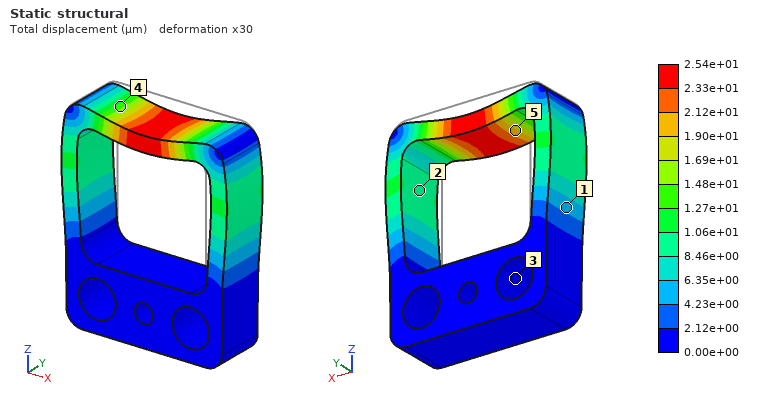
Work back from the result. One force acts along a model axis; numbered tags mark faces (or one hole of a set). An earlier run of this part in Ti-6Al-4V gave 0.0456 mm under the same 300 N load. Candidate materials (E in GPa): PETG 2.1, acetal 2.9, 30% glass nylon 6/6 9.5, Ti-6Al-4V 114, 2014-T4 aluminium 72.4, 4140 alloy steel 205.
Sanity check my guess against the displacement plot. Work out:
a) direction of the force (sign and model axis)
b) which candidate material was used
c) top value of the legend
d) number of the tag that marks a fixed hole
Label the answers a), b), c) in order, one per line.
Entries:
a) -Z
b) 4140 alloy steel
c) 2.54e+01 µm
d) 3
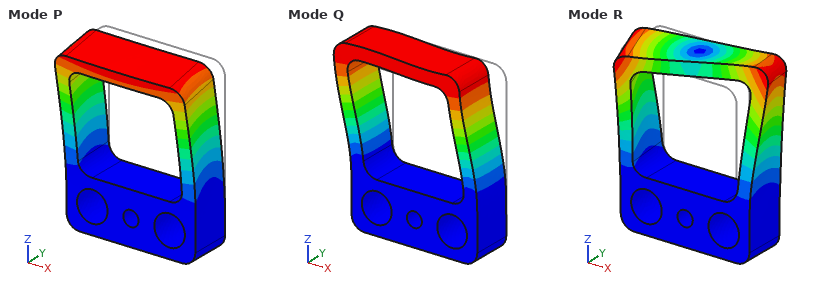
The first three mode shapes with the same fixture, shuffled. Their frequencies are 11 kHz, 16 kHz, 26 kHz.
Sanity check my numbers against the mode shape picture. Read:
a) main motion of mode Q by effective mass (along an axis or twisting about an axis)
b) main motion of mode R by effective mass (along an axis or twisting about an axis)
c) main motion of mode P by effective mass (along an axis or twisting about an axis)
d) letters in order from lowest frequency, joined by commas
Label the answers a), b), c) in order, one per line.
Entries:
a) along X
b) twisting about Z
c) along Y
d) Q, P, R
